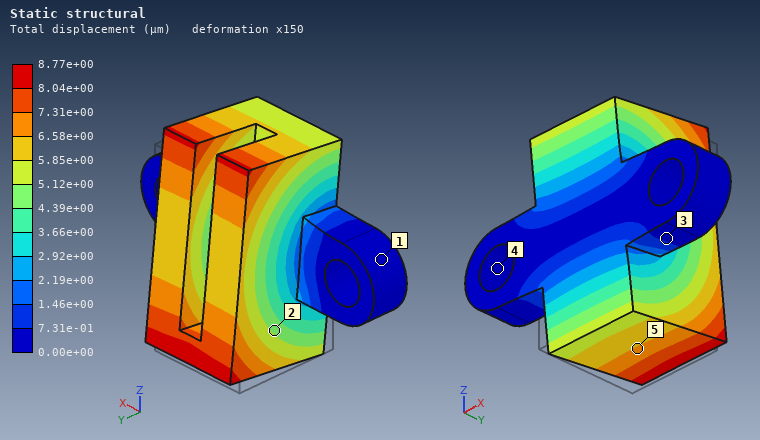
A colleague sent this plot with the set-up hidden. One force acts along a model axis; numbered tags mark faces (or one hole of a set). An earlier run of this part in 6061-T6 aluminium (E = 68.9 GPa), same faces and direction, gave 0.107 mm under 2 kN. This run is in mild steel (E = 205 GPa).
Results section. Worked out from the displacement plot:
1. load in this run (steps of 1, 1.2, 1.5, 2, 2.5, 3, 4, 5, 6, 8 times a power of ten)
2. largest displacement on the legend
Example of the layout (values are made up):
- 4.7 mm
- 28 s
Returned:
- 500 N
- 8.77e+00 µm
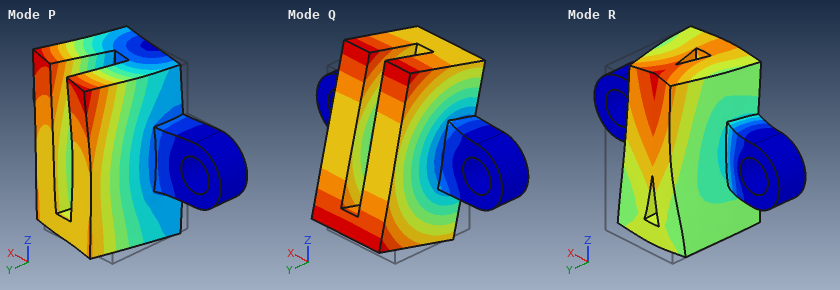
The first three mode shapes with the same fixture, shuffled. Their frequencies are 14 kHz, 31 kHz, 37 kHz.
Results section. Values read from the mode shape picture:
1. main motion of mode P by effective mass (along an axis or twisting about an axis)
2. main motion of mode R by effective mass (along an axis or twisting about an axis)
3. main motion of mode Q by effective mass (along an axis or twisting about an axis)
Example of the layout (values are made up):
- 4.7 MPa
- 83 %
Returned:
- along X
- along Y
- along Z
